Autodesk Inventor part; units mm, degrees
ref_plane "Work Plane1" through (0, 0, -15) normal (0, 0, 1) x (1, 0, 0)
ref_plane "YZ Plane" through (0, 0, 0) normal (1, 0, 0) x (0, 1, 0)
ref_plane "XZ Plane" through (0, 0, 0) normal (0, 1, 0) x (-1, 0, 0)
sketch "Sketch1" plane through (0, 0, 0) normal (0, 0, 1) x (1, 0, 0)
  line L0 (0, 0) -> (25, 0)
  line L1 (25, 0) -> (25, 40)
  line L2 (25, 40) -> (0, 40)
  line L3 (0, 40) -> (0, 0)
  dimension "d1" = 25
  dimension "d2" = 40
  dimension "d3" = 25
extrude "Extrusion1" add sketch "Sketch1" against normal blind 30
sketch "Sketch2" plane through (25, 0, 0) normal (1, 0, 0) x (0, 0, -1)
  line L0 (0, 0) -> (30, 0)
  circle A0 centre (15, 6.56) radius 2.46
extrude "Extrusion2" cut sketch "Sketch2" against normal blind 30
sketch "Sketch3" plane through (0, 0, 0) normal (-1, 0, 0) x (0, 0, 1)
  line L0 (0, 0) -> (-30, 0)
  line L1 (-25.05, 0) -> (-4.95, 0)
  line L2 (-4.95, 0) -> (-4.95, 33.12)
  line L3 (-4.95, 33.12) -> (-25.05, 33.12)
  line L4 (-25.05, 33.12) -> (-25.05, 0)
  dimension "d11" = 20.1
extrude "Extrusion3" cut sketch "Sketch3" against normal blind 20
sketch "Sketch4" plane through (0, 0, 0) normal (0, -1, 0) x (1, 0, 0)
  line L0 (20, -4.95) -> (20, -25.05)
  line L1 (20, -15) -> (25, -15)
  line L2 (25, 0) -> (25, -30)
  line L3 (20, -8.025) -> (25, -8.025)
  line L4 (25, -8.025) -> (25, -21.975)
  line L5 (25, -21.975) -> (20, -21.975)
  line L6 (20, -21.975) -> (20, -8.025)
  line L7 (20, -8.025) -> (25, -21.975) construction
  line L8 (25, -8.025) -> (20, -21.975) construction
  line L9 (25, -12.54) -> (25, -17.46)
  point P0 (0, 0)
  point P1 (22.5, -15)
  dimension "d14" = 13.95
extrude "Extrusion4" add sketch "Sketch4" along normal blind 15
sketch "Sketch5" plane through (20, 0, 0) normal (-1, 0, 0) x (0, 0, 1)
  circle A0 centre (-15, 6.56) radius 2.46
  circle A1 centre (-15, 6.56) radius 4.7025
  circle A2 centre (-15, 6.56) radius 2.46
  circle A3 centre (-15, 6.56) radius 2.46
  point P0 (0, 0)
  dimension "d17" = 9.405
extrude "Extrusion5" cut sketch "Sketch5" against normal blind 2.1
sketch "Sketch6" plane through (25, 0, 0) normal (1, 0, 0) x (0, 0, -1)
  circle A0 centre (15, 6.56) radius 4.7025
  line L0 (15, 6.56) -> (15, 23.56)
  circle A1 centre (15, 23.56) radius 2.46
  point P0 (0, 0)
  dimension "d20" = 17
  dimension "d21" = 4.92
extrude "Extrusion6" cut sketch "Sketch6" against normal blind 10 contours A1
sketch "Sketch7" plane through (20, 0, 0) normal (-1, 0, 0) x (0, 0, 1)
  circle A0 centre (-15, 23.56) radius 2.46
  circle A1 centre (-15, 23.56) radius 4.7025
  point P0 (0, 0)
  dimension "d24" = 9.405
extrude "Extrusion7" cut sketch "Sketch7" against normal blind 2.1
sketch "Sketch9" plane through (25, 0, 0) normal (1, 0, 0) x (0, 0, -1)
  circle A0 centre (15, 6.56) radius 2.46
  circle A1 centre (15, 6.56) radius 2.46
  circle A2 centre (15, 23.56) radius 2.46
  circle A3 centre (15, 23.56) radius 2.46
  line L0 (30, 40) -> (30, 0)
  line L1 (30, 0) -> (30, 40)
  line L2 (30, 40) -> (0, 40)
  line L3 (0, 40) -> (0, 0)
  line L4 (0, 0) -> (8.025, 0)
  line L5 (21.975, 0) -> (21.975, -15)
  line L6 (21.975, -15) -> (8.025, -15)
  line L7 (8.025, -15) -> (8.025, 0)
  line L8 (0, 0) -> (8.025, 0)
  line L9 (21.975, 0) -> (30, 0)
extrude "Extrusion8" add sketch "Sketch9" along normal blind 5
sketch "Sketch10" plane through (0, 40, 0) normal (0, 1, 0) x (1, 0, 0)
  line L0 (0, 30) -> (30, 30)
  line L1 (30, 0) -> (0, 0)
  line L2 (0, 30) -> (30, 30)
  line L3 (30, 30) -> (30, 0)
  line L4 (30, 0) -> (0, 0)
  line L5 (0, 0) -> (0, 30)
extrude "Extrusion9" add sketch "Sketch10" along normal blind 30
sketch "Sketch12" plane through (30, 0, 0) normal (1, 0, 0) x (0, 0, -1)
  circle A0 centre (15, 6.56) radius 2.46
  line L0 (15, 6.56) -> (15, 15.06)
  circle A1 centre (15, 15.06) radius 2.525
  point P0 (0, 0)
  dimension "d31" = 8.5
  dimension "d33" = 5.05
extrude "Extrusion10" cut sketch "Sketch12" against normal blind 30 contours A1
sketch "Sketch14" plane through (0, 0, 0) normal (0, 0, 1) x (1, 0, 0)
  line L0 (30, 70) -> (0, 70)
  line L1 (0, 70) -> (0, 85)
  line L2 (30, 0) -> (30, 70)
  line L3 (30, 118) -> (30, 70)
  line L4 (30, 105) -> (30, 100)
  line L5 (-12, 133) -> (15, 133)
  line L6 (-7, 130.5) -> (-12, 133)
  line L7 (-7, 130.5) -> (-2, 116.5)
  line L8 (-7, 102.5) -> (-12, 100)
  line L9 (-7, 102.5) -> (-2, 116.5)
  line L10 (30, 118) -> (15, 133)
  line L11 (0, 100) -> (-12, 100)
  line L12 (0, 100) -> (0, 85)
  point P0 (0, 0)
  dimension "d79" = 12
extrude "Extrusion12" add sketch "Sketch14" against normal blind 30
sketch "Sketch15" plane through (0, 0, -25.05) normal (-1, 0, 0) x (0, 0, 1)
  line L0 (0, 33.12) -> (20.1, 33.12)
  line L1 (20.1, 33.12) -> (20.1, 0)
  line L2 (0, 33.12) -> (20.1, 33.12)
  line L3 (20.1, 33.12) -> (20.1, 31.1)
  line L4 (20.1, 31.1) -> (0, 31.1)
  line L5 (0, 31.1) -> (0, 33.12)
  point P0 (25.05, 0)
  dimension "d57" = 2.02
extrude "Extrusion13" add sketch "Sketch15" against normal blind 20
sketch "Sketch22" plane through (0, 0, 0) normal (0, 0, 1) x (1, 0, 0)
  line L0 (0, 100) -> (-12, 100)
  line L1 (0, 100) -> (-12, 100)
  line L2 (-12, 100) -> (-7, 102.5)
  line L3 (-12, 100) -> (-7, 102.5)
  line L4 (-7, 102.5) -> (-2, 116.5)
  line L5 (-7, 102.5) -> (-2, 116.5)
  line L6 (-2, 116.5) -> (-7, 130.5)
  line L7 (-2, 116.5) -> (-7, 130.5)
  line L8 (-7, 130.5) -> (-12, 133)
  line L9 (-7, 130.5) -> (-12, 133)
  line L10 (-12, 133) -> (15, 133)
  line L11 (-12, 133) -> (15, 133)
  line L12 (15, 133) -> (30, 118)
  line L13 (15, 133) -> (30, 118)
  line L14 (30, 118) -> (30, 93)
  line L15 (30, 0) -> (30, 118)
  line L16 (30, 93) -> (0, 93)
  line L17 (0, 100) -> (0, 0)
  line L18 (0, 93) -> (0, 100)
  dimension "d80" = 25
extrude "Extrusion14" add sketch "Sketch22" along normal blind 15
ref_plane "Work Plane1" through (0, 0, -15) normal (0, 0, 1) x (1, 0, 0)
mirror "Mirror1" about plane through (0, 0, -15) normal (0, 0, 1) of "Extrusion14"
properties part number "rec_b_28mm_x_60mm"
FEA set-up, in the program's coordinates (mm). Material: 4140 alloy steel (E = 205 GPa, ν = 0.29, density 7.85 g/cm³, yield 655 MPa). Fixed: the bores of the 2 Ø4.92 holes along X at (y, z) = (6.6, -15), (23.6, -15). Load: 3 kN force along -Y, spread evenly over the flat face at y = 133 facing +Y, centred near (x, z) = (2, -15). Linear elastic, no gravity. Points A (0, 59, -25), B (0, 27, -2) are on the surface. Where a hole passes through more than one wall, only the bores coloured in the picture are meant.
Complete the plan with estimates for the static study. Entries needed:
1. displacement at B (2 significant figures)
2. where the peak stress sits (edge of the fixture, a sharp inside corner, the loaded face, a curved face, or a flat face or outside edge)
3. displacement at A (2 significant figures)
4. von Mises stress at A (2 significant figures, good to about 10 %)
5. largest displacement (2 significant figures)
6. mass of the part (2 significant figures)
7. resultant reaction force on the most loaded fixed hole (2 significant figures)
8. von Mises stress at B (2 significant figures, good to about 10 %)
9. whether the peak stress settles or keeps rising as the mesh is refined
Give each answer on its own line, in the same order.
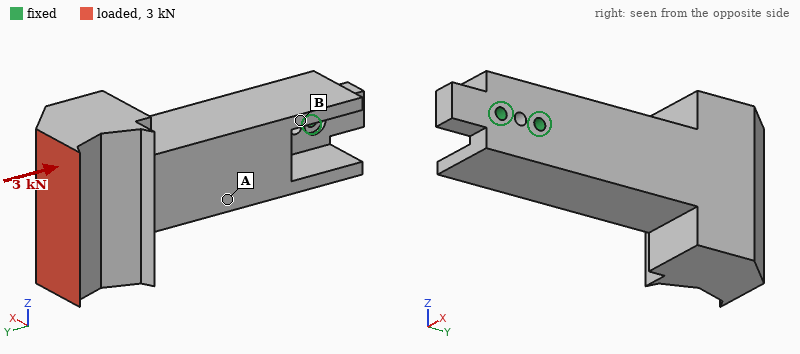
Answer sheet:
13 µm
edge of the fixture
25 µm
13 MPa
79 µm
1.2 kg
3.4 kN
29 MPa
keeps rising
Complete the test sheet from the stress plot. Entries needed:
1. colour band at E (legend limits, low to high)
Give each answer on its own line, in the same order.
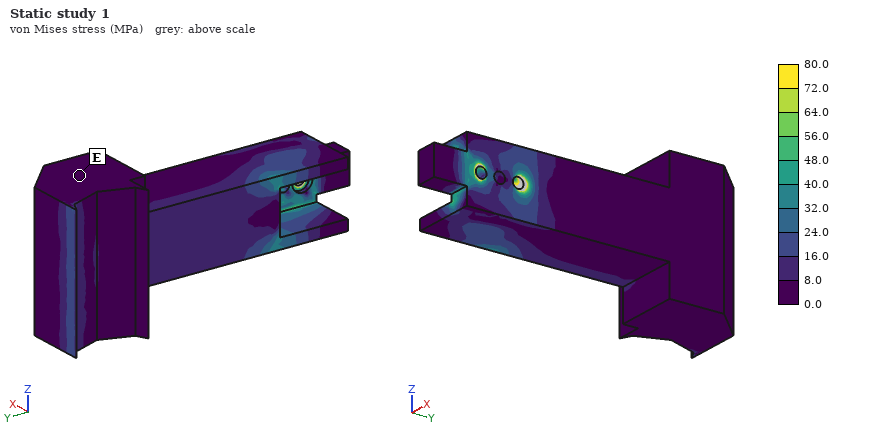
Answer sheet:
0.0 to 8.0 MPa
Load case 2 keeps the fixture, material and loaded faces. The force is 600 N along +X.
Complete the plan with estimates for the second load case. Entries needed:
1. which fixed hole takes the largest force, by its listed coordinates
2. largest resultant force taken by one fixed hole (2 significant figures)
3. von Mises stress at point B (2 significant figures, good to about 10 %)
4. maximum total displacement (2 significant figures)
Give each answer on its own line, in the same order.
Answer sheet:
(23.6, -15)
3.2 kN
27 MPa
74 µm
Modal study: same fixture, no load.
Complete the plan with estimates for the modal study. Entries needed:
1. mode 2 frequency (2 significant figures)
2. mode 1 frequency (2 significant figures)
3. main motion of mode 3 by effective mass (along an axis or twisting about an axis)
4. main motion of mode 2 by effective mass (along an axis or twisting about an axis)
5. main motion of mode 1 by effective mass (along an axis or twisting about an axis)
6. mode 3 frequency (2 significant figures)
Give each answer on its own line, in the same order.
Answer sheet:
810 Hz
690 Hz
twisting about Y
along Z
along X
1900 Hz
